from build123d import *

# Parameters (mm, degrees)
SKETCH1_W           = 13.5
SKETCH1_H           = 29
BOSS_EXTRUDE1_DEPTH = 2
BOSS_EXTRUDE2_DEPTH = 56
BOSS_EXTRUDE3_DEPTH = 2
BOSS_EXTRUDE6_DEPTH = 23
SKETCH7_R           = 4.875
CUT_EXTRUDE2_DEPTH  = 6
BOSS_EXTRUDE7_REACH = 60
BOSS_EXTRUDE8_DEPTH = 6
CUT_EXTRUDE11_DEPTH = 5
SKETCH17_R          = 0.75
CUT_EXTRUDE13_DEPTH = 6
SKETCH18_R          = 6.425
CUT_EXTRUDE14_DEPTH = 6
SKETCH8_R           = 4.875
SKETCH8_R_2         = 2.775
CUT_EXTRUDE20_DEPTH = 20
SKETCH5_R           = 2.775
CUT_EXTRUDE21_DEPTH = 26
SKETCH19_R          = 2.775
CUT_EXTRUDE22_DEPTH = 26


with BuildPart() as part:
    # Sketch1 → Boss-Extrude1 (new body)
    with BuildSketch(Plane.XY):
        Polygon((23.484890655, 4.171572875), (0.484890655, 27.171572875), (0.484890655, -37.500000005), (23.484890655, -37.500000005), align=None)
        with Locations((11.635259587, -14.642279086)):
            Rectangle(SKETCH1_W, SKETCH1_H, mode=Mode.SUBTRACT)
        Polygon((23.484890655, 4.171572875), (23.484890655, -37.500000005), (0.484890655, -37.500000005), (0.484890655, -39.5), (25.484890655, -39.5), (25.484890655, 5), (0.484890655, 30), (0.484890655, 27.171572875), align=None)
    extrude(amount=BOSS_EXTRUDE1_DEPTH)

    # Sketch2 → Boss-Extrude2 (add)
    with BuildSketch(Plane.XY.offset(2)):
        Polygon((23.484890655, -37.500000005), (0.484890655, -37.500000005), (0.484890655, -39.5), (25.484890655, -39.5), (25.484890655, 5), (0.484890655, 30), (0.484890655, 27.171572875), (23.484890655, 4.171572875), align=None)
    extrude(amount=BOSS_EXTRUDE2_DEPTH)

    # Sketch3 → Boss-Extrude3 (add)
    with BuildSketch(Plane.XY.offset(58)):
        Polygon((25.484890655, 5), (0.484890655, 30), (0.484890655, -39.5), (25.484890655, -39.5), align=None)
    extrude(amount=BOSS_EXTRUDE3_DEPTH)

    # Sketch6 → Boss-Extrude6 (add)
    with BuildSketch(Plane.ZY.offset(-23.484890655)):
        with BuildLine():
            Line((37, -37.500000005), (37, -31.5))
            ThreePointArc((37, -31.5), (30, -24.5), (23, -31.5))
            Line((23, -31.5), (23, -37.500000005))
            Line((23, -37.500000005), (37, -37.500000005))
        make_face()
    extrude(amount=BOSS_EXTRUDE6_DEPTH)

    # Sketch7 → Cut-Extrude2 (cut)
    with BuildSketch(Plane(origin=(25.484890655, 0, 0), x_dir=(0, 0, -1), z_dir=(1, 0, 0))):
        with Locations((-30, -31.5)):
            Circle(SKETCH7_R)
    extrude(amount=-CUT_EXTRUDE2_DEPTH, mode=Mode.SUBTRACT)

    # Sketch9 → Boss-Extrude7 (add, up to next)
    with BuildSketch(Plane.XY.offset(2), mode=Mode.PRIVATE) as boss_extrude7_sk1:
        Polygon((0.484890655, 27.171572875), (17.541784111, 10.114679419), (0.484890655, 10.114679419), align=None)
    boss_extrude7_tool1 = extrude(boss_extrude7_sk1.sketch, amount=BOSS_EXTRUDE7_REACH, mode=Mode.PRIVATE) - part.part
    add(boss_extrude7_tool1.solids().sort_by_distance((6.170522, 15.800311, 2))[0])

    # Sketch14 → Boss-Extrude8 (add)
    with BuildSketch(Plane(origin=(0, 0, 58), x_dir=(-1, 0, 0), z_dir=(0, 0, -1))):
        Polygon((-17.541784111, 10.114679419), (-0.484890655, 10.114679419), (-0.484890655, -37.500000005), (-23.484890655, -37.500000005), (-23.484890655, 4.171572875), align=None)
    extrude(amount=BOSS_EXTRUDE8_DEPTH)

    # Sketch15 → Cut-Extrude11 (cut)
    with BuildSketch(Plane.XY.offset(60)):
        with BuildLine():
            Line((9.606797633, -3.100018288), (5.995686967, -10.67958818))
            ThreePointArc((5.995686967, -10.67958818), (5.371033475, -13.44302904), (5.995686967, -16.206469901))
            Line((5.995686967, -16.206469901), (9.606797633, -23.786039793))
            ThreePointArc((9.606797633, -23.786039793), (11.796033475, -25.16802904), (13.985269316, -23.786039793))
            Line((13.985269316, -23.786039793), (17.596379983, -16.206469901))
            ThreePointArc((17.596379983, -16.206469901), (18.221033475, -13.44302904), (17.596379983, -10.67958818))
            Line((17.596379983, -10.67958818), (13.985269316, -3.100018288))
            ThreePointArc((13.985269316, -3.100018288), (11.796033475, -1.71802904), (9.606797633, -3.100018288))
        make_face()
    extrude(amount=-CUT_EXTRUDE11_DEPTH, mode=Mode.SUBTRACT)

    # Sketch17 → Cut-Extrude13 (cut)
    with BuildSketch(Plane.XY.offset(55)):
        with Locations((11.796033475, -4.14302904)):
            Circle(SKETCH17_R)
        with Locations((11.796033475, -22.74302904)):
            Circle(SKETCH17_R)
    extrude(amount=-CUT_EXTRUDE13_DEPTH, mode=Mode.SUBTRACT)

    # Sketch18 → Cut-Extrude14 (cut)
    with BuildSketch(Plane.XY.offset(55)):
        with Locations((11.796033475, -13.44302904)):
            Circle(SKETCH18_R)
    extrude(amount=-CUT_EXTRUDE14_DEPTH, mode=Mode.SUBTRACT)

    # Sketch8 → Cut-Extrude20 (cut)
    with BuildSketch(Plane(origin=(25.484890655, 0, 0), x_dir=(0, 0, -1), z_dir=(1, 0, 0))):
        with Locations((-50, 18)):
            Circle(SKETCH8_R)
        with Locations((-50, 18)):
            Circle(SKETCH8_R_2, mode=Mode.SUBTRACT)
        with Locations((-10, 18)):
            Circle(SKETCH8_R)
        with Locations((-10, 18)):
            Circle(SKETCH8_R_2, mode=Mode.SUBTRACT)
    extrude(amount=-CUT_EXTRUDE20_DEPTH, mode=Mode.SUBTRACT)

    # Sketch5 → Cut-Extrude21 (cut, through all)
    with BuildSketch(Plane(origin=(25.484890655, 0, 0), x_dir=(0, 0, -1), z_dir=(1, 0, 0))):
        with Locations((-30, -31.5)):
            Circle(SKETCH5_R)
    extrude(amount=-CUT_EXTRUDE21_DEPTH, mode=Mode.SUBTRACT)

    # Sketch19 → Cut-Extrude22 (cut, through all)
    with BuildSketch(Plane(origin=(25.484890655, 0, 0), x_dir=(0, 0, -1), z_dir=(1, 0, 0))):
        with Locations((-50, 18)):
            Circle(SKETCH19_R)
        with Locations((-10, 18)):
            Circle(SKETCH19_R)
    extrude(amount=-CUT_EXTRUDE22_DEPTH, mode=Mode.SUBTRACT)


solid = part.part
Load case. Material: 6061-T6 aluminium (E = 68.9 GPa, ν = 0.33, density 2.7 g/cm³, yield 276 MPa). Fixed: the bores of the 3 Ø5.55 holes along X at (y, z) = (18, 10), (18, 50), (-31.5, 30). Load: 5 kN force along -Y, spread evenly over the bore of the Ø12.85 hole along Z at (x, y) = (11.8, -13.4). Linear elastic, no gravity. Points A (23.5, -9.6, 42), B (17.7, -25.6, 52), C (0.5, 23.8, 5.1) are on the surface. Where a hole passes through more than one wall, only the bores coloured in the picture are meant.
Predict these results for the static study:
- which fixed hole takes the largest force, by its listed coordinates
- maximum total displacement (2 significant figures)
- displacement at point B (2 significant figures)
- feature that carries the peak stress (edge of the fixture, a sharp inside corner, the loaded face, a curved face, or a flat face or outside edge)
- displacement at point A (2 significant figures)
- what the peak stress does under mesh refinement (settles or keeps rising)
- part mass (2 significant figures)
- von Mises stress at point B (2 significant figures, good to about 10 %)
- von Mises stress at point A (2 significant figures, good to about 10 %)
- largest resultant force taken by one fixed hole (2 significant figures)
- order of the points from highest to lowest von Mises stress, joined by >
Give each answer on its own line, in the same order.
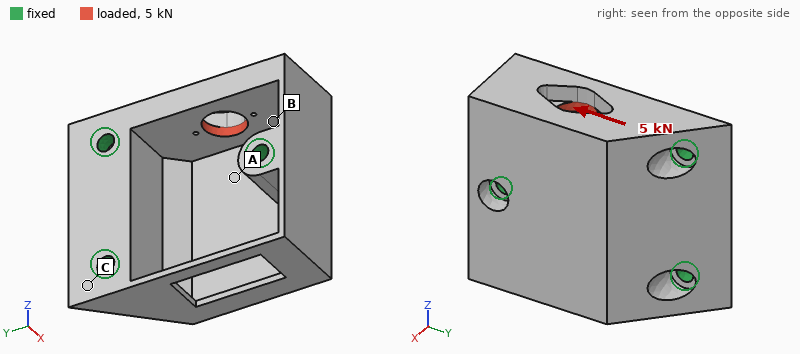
(18, 50)
38 µm
29 µm
edge of the fixture
19 µm
keeps rising
84 g
28 MPa
21 MPa
3.8 kN
B > A > C
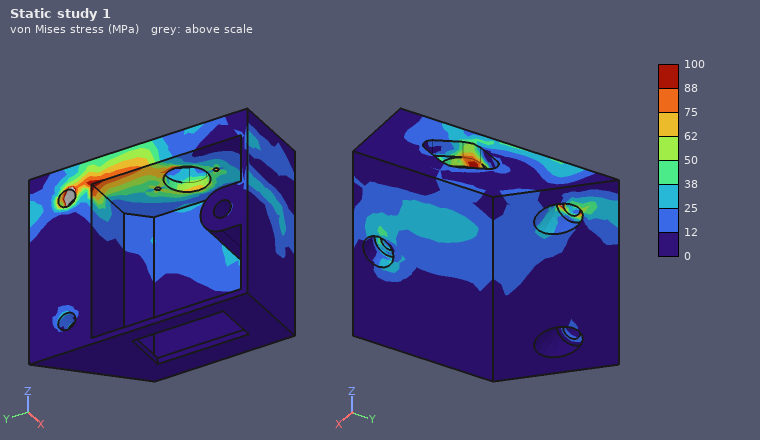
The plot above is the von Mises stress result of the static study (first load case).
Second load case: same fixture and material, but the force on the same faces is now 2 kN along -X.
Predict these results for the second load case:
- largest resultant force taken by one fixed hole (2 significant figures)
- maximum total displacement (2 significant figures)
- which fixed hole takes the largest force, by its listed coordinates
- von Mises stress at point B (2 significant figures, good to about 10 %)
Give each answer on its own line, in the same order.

1.5 kN
34 µm
(18, 50)
19 MPa
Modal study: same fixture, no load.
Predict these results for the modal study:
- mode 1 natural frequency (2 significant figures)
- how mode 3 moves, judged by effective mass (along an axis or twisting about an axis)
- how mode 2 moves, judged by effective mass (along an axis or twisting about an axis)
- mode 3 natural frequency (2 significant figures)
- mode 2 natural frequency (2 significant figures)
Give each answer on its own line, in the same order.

5300 Hz
along X
along X
8700 Hz
7700 Hz
